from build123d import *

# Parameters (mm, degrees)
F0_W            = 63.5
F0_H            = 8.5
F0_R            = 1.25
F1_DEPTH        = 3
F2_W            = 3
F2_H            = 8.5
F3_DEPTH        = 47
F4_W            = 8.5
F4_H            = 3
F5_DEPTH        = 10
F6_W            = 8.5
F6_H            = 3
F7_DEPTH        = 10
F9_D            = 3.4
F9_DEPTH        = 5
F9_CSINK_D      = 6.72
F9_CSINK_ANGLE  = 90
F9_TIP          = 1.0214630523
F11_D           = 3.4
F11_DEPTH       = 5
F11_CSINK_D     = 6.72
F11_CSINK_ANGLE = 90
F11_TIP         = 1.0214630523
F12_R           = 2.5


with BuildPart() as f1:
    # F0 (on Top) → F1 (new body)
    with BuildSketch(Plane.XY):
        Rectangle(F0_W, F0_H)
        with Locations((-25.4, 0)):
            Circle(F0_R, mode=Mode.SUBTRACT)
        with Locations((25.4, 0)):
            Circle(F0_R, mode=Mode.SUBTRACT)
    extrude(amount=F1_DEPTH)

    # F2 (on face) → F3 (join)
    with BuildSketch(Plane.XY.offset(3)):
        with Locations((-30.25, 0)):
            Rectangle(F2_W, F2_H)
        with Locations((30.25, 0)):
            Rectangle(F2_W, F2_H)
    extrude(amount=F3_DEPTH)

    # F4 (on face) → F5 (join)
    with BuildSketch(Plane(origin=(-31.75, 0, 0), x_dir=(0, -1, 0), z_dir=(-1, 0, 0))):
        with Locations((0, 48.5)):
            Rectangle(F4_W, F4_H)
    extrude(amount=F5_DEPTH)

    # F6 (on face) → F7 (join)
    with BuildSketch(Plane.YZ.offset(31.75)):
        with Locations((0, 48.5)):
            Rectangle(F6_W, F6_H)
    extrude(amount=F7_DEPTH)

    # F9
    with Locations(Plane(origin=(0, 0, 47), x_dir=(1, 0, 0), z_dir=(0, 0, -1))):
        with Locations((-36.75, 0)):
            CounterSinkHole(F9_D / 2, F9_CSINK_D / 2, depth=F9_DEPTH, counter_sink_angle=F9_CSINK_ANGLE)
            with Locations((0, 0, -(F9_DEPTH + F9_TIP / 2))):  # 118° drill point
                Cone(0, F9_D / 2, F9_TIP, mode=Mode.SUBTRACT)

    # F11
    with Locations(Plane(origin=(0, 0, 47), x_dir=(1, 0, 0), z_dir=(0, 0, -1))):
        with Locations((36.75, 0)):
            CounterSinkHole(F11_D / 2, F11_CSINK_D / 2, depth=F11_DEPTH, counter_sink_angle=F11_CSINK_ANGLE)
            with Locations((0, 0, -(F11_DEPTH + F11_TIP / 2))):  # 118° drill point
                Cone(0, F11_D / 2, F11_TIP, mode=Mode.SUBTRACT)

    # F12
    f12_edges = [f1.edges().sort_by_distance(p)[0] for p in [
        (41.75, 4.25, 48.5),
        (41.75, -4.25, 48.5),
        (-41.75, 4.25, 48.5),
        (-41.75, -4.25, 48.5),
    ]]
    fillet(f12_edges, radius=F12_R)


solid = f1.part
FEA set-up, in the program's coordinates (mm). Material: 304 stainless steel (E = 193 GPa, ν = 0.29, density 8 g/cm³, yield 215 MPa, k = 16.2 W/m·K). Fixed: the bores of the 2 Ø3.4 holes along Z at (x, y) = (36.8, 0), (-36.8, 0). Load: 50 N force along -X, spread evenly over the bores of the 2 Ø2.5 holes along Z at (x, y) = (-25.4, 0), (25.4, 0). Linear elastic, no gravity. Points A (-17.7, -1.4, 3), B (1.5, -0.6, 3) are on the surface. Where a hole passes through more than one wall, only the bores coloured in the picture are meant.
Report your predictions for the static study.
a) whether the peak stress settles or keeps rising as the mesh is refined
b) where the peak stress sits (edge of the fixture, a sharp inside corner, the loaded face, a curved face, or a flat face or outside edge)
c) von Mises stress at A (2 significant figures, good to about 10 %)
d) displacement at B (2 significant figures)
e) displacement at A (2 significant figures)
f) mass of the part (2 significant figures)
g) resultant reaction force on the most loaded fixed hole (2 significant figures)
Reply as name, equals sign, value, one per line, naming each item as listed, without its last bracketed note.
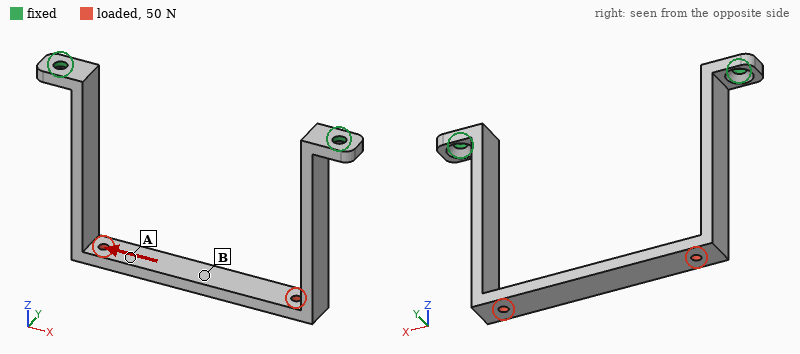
whether the peak stress settles or keeps rising as the mesh is refined = keeps rising
where the peak stress sits = edge of the fixture
von Mises stress at A = 26 MPa
displacement at B = 0.12 mm
displacement at A = 0.12 mm
mass of the part = 35 g
resultant reaction force on the most loaded fixed hole = 31 N
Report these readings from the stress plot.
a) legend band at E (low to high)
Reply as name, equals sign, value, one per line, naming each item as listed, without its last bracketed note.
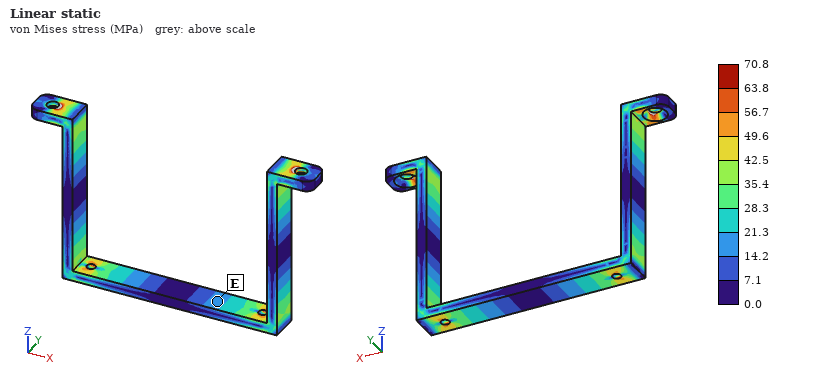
legend band at E = 14.2 to 21.3 MPa
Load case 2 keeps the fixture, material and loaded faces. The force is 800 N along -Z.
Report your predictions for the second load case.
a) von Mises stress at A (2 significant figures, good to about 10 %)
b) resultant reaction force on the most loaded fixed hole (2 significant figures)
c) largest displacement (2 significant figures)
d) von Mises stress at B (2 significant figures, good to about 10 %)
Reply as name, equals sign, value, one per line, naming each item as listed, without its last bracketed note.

von Mises stress at A = 39 MPa
resultant reaction force on the most loaded fixed hole = 400 N
largest displacement = 79 µm
von Mises stress at B = 41 MPa
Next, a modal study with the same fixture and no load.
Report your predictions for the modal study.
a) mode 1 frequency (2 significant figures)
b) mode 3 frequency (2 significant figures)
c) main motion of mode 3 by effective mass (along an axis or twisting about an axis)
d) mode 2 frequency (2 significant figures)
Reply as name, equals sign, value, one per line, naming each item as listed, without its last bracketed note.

mode 1 frequency = 750 Hz
mode 3 frequency = 1400 Hz
main motion of mode 3 by effective mass = twisting about Z
mode 2 frequency = 770 Hz
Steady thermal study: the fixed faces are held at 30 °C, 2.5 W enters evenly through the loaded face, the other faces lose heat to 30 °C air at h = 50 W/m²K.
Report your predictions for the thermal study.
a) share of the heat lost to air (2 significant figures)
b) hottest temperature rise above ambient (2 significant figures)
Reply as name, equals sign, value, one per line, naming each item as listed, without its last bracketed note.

share of the heat lost to air = 95 %
hottest temperature rise above ambient = 31 K
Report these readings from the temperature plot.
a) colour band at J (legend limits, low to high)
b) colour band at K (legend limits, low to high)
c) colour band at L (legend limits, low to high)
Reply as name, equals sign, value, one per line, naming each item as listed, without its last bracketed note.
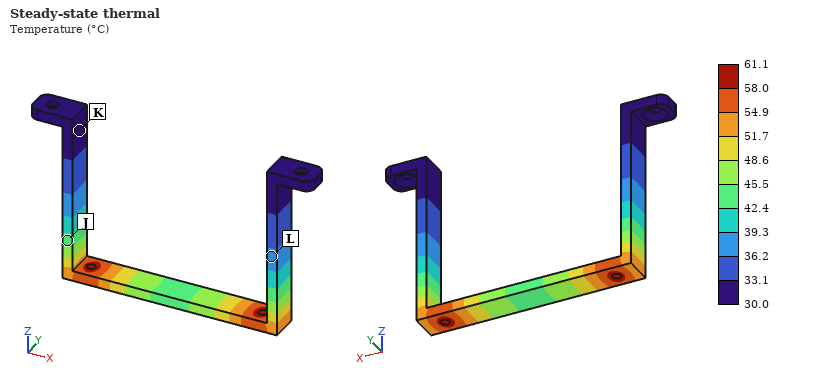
colour band at J = 42.4 to 45.5 °C
colour band at K = 30.0 to 33.1 °C
colour band at L = 36.2 to 39.3 °C
